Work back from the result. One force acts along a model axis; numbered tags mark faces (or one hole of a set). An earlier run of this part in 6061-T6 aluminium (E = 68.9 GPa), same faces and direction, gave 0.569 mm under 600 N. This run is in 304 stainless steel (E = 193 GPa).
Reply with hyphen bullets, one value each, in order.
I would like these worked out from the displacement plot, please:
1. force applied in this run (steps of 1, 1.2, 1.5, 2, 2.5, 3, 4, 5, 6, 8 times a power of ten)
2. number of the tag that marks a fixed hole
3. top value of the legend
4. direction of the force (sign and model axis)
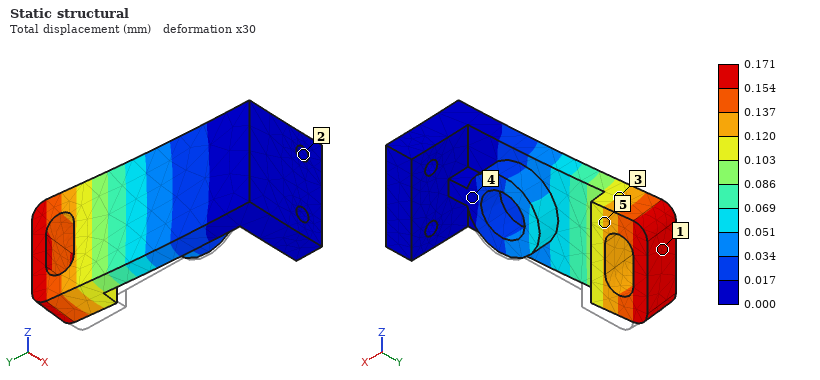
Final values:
- 500 N
- 2
- 0.171 mm
- -X
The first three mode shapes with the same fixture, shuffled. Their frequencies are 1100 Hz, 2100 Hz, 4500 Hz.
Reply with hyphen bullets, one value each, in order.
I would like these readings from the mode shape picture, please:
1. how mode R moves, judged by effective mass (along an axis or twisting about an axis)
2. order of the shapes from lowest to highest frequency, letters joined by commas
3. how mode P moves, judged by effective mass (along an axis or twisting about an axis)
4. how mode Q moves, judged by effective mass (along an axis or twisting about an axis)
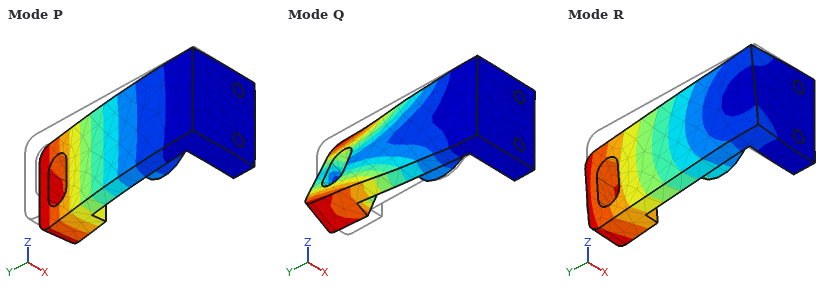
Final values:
- along Z
- P, R, Q
- along X
- twisting about Y
